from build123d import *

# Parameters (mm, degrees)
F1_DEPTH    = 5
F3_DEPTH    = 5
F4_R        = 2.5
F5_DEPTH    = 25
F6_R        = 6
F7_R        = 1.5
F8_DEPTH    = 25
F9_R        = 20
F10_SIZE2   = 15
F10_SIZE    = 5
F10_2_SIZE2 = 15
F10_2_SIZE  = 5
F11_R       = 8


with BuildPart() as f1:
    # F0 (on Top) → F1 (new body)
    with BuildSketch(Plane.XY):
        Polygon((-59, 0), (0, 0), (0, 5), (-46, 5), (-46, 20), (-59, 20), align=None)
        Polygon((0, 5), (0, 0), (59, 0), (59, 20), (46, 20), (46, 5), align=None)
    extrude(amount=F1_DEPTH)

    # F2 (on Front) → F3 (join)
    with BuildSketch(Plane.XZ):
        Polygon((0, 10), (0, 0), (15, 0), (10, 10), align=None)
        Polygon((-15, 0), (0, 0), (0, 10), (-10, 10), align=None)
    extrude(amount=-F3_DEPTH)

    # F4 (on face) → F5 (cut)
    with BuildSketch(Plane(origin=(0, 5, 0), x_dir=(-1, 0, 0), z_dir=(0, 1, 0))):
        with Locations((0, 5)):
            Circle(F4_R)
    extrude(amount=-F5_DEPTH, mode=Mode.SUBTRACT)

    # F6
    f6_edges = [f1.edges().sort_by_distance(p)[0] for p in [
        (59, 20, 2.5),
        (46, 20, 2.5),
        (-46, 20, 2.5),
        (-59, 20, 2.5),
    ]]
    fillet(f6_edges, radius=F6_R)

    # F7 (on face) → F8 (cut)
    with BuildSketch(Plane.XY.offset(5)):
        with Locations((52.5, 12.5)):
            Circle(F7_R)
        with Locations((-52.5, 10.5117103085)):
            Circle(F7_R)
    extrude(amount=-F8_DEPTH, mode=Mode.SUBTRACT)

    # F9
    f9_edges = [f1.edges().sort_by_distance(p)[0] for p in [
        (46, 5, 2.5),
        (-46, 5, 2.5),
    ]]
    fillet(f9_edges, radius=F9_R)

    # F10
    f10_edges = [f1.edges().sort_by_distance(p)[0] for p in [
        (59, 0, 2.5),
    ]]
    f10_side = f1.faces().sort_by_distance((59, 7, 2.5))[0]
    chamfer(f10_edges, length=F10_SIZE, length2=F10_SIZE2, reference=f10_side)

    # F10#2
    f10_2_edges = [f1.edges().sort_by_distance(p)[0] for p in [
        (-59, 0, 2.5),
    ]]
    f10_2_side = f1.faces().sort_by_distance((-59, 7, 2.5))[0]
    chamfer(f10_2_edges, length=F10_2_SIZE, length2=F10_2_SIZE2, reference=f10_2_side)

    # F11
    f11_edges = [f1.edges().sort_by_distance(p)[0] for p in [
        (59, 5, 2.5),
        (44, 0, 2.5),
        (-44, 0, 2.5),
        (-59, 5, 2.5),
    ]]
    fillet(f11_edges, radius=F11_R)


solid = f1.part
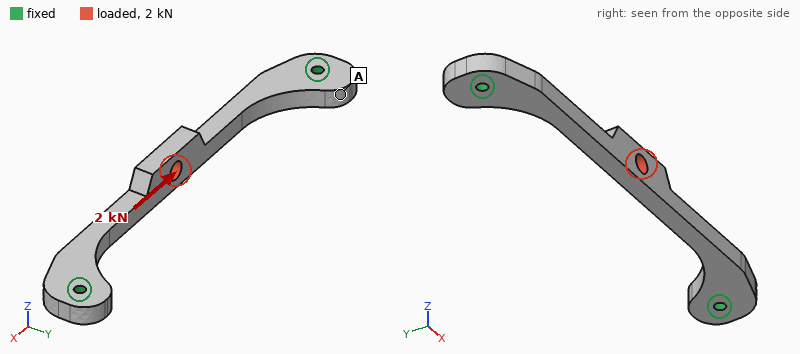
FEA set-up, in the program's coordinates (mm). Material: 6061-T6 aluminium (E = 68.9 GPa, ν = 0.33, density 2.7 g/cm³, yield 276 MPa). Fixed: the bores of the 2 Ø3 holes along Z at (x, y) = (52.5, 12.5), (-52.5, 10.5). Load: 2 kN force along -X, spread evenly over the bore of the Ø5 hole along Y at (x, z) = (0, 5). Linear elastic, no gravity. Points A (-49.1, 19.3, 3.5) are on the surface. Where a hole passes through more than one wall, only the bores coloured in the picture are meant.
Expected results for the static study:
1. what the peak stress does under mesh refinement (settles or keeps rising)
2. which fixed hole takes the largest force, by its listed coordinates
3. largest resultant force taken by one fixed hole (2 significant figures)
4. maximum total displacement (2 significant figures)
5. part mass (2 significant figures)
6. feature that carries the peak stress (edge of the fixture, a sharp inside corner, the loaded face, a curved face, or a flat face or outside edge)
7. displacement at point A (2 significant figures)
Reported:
keeps rising
(-52.5, 10.5)
1.1 kN
89 µm
14 g
edge of the fixture
15 µm
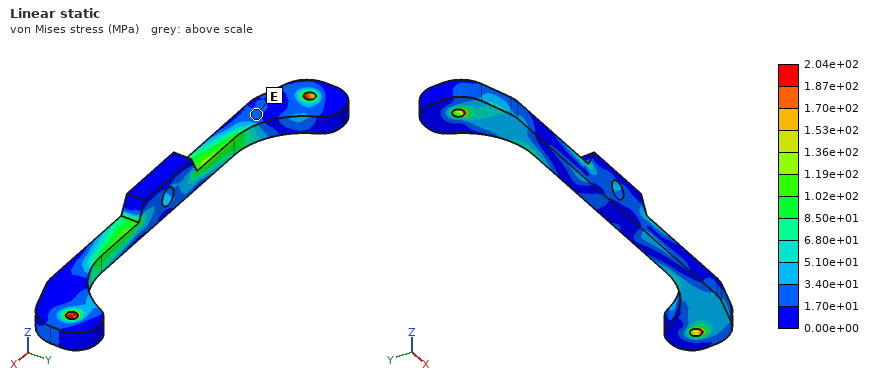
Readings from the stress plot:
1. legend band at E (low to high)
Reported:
1.70e+01 to 3.40e+01 MPa
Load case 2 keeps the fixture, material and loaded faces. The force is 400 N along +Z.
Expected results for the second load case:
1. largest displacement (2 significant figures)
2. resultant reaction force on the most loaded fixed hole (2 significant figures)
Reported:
0.32 mm
220 N
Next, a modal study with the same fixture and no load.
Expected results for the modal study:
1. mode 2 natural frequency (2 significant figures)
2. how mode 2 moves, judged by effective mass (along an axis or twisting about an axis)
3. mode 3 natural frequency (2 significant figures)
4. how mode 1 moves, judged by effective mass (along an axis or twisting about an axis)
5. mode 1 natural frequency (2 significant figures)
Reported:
3400 Hz
along Y
6500 Hz
along Z
2700 Hz
